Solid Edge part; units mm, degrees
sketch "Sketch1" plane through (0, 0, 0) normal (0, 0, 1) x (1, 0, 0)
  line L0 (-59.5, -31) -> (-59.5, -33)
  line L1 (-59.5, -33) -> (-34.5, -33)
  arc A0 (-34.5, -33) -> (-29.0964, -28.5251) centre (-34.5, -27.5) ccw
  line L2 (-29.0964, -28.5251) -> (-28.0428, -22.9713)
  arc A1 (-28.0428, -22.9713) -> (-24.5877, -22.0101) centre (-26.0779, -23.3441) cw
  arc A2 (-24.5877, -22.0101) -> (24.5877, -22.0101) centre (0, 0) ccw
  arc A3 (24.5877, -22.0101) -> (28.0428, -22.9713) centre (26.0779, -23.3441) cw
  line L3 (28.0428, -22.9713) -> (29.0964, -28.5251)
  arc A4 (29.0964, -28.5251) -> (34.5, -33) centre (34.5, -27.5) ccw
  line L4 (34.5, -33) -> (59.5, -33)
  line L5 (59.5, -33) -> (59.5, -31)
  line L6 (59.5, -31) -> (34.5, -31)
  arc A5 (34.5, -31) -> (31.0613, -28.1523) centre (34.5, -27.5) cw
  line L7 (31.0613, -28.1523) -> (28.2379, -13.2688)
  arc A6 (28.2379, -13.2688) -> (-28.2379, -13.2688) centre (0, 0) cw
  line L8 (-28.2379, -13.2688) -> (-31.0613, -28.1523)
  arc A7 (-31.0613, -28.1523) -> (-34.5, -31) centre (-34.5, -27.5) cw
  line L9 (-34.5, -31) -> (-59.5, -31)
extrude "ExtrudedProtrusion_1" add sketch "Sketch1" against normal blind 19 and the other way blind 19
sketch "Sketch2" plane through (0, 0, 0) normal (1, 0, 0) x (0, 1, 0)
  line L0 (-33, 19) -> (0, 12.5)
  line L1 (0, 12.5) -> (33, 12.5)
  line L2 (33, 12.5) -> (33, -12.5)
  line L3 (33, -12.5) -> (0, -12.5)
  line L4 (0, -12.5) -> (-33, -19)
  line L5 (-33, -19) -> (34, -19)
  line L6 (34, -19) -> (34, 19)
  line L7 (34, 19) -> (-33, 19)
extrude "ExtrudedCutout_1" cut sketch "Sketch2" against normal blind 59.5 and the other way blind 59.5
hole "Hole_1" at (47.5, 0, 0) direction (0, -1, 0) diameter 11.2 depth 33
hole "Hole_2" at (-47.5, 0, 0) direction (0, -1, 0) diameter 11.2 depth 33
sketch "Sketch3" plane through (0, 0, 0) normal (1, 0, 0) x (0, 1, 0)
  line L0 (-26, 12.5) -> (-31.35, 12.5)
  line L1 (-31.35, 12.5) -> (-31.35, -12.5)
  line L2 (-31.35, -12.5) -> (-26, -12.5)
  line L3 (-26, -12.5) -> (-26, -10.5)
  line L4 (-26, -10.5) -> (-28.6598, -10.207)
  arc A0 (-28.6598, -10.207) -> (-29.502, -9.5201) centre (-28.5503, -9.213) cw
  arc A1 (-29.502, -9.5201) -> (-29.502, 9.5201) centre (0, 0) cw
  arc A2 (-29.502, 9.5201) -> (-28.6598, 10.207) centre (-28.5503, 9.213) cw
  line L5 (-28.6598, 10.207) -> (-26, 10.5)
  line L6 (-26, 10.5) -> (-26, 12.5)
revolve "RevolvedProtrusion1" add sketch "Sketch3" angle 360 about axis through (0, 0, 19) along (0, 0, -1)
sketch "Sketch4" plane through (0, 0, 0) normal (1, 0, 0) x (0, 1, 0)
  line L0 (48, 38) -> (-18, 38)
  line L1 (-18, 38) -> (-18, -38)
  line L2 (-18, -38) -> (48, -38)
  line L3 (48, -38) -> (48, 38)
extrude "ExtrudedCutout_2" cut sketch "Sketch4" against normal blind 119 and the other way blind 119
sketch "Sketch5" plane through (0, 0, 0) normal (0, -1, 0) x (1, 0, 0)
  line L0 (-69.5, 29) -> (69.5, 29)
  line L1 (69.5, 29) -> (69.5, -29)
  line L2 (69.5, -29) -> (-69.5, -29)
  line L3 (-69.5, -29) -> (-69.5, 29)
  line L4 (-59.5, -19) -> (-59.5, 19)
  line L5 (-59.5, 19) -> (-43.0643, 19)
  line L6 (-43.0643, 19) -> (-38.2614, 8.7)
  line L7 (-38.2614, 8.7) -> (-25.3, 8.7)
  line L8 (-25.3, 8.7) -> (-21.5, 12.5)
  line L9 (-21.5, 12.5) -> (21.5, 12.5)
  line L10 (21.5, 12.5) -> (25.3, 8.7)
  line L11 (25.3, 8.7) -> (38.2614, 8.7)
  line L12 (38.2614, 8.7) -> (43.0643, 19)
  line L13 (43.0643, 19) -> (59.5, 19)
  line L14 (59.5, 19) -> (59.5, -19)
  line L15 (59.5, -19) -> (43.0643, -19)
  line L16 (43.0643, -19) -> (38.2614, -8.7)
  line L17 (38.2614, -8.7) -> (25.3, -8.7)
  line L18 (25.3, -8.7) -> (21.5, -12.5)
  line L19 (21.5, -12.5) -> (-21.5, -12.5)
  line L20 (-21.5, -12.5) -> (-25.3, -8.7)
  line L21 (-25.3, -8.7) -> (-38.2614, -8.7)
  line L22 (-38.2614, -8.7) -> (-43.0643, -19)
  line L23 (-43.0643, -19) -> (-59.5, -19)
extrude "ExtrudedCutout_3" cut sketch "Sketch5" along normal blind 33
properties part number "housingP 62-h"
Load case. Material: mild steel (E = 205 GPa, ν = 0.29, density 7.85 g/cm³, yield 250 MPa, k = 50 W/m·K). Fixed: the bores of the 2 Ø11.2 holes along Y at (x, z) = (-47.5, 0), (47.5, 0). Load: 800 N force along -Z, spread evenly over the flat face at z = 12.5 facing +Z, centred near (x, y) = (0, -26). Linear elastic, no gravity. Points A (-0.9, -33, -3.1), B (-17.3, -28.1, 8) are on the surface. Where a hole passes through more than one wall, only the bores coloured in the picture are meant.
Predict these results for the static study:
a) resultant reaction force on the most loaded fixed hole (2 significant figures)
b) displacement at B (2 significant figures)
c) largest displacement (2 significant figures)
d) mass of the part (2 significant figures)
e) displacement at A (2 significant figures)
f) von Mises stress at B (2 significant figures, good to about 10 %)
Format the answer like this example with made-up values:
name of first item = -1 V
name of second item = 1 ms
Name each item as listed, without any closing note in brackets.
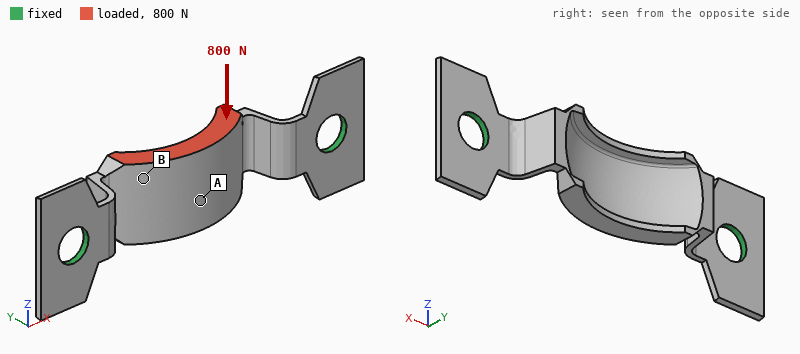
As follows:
resultant reaction force on the most loaded fixed hole = 400 N
displacement at B = 42 µm
largest displacement = 66 µm
mass of the part = 70 g
displacement at A = 32 µm
von Mises stress at B = 33 MPa
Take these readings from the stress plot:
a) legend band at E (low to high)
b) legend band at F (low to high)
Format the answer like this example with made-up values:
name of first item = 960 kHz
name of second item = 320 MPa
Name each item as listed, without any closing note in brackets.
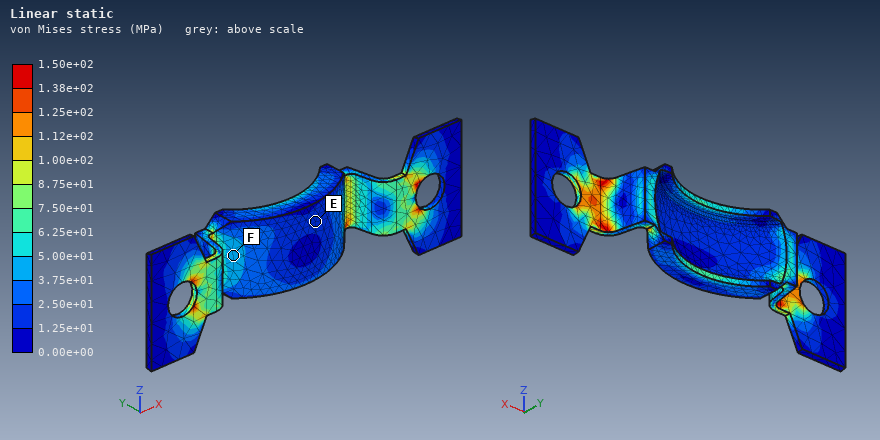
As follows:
legend band at E = 1.25e+01 to 2.50e+01 MPa
legend band at F = 3.75e+01 to 5.00e+01 MPa
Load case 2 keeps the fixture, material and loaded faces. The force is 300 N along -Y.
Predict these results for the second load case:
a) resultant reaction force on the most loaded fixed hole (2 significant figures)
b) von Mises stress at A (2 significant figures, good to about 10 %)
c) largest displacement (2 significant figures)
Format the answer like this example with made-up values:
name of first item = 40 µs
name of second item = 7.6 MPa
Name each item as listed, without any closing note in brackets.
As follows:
resultant reaction force on the most loaded fixed hole = 200 N
von Mises stress at A = 20 MPa
largest displacement = 0.12 mm
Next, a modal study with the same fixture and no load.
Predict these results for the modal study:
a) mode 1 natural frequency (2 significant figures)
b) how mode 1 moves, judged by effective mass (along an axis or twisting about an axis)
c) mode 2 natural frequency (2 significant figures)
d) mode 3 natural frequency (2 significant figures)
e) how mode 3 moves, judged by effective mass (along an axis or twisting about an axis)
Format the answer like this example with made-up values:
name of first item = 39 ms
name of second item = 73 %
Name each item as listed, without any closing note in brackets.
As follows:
mode 1 natural frequency = 2200 Hz
how mode 1 moves, judged by effective mass = along Y
mode 2 natural frequency = 2300 Hz
mode 3 natural frequency = 2500 Hz
how mode 3 moves, judged by effective mass = along X
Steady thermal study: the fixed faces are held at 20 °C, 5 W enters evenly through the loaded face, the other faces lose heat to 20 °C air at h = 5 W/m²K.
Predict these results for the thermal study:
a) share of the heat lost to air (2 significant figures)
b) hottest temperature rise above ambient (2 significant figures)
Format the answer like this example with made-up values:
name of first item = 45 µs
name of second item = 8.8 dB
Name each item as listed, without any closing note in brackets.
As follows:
share of the heat lost to air = 16 %
hottest temperature rise above ambient = 45 K
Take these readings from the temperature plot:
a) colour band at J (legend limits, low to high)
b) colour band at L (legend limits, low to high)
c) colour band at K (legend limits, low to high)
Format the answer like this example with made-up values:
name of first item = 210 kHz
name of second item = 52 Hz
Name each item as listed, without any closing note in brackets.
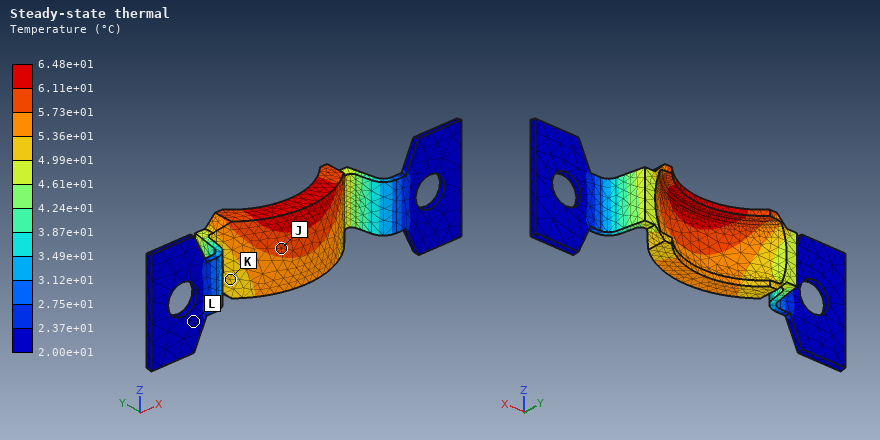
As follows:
colour band at J = 5.73e+01 to 6.11e+01 °C
colour band at L = 2.00e+01 to 2.37e+01 °C
colour band at K = 4.99e+01 to 5.36e+01 °C
